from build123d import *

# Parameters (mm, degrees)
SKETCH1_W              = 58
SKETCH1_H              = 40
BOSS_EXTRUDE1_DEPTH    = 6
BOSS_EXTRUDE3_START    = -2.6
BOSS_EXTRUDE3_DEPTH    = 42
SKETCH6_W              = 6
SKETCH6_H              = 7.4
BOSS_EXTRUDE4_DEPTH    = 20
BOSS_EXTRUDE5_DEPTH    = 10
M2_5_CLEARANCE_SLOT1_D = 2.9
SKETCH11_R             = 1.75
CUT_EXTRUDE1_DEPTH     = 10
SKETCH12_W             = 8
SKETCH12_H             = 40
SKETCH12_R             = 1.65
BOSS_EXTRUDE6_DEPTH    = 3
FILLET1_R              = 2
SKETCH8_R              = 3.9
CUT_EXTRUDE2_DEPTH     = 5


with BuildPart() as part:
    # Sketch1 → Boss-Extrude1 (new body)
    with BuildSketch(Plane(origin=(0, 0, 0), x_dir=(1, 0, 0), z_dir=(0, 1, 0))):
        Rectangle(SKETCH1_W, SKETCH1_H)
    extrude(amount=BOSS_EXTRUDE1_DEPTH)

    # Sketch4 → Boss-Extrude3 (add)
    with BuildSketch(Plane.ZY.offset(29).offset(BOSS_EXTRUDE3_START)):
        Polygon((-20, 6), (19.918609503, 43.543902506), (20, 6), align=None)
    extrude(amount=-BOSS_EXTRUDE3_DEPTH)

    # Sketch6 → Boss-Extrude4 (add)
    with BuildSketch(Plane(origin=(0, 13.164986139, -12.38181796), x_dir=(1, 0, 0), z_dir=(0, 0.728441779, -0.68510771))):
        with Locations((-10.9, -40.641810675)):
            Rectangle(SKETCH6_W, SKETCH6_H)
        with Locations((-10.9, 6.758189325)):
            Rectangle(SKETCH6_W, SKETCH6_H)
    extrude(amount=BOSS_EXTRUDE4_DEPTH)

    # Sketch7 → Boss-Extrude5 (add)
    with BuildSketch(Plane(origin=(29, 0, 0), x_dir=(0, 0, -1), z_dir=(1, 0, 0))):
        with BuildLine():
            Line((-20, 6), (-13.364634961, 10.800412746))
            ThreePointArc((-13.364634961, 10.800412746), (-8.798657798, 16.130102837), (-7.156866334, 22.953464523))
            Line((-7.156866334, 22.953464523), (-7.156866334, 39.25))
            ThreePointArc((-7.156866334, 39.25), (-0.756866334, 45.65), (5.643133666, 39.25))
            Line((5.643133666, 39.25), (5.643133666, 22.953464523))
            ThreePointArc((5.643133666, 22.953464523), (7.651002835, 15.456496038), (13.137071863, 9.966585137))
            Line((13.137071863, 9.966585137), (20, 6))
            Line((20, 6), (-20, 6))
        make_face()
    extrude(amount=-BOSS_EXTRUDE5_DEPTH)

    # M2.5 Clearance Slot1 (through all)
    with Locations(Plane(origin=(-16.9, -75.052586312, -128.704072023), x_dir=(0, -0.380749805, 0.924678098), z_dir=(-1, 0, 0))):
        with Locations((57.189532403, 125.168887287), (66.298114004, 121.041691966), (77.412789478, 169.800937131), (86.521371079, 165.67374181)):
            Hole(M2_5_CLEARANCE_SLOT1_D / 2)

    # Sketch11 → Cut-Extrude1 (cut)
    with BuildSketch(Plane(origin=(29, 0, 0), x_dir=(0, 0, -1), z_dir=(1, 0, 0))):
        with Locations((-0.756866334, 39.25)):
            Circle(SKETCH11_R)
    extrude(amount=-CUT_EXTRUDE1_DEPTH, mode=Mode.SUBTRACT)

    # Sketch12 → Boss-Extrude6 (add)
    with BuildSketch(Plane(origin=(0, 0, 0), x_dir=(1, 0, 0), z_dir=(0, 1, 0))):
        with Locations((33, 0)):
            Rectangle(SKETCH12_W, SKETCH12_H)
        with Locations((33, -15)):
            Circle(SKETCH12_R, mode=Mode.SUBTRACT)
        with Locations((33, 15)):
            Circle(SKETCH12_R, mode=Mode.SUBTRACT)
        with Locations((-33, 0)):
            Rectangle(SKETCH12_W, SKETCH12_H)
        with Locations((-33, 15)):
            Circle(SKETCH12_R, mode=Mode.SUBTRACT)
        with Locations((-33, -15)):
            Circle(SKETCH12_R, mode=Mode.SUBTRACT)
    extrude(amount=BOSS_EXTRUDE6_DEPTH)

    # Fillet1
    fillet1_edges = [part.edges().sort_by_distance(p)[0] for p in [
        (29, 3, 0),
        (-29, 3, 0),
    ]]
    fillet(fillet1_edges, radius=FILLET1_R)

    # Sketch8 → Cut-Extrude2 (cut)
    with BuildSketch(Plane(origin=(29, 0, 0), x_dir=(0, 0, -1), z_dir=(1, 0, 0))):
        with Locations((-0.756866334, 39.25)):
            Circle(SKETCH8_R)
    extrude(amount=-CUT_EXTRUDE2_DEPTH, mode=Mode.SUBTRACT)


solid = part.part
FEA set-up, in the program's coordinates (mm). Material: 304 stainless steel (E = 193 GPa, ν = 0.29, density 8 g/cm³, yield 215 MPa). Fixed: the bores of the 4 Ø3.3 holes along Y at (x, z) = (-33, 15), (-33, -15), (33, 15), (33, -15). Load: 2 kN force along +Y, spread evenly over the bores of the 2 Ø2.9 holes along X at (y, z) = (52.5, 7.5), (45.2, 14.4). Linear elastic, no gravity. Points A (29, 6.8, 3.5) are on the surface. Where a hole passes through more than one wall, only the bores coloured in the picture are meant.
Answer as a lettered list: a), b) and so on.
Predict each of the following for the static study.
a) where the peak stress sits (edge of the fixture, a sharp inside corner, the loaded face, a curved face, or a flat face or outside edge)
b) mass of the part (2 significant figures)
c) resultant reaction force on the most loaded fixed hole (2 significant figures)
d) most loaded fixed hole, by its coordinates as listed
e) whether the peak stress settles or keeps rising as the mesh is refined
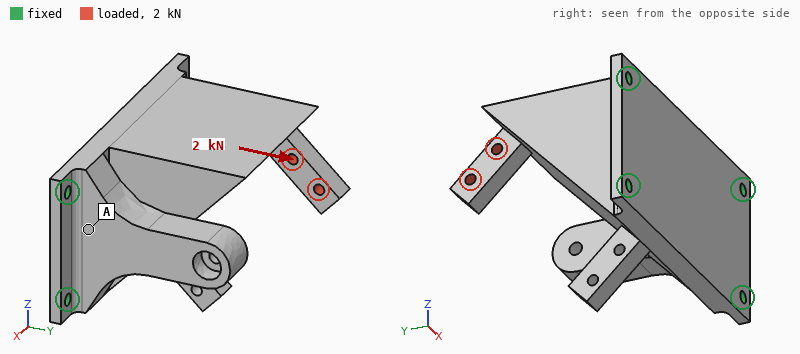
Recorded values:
a) edge of the fixture
b) 440 g
c) 1.4 kN
d) (-33, 15)
e) keeps rising
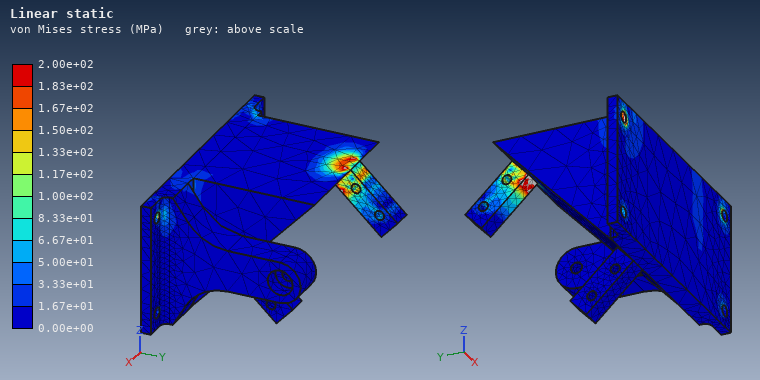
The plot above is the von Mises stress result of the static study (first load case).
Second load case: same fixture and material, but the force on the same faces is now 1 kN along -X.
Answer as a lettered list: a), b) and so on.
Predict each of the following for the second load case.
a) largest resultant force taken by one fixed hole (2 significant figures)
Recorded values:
a) 620 N
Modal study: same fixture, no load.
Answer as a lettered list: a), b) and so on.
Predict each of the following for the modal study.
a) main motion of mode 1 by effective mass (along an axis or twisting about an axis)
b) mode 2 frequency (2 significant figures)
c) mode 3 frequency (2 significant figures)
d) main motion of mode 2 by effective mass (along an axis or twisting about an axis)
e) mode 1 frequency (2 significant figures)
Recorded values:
a) along Y
b) 4000 Hz
c) 6000 Hz
d) along Z
e) 3300 Hz
